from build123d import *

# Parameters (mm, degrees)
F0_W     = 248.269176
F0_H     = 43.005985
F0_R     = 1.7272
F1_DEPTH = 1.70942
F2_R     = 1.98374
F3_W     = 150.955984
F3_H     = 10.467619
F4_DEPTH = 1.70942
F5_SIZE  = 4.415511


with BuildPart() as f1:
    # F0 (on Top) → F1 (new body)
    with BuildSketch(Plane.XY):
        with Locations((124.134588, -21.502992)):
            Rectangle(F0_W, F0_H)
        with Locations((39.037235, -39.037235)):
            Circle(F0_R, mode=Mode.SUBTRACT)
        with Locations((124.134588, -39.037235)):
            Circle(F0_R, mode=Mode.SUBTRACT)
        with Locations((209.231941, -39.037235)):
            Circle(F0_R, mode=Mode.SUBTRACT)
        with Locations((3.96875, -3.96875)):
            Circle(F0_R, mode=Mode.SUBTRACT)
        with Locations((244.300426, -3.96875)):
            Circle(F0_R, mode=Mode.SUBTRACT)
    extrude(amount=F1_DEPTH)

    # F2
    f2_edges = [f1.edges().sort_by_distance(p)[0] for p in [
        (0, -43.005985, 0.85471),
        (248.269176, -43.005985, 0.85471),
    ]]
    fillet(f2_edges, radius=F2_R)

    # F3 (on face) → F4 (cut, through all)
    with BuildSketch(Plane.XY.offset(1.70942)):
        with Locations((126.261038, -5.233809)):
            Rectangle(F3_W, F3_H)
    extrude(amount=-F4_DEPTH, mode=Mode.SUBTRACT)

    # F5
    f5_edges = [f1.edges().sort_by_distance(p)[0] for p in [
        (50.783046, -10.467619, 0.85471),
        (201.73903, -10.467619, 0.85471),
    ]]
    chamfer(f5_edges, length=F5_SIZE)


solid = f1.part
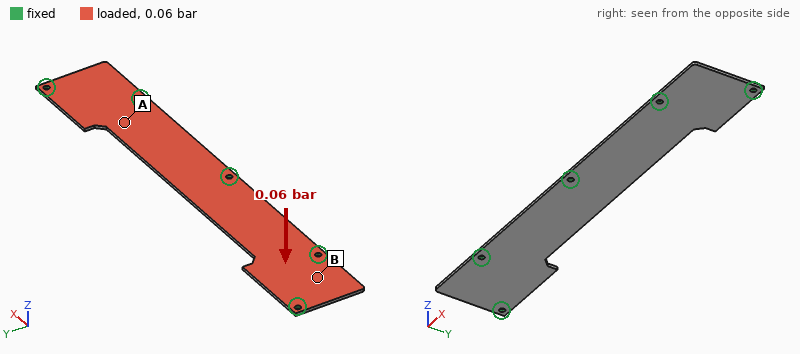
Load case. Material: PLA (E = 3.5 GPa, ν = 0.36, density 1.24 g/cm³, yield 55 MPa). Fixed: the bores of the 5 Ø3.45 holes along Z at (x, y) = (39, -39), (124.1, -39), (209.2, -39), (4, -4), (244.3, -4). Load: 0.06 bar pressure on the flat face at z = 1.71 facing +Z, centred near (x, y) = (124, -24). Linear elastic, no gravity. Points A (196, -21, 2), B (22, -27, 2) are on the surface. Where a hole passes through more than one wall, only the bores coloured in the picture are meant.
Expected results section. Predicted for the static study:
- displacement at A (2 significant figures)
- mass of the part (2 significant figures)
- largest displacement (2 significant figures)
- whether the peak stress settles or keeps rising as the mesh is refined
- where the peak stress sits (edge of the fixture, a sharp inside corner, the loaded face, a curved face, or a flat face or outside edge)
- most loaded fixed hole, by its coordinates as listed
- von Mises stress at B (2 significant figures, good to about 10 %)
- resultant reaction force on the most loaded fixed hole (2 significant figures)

0.57 mm
19 g
1.3 mm
keeps rising
edge of the fixture
(124.1, -39)
2.6 MPa
17 N
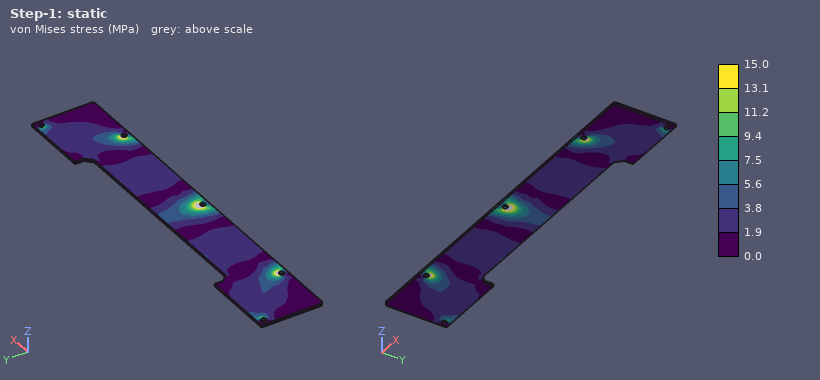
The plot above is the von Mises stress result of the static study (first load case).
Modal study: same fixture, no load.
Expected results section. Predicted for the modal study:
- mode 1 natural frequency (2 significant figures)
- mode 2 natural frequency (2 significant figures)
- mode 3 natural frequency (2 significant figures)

300 Hz
300 Hz
530 Hz
